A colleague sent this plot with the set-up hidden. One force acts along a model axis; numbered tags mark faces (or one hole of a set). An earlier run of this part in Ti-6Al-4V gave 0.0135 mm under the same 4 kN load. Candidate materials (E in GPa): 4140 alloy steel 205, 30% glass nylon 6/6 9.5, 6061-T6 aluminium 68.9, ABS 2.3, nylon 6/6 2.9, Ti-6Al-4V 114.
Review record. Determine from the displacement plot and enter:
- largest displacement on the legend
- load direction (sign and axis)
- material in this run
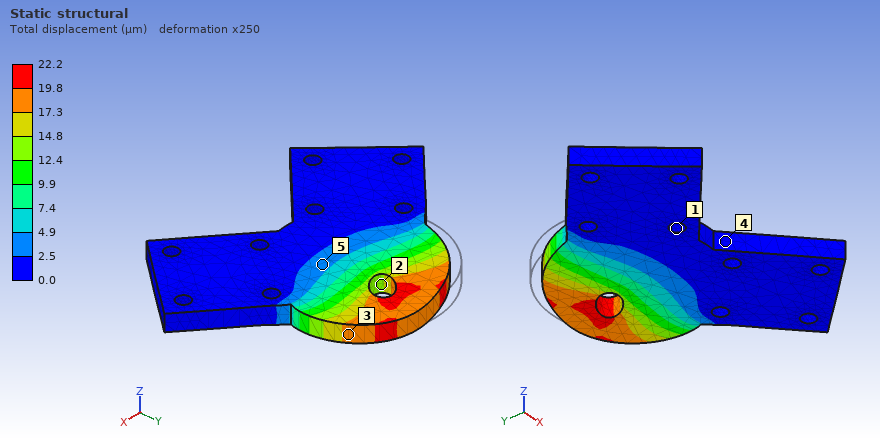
22.2 µm
+X
6061-T6 aluminium
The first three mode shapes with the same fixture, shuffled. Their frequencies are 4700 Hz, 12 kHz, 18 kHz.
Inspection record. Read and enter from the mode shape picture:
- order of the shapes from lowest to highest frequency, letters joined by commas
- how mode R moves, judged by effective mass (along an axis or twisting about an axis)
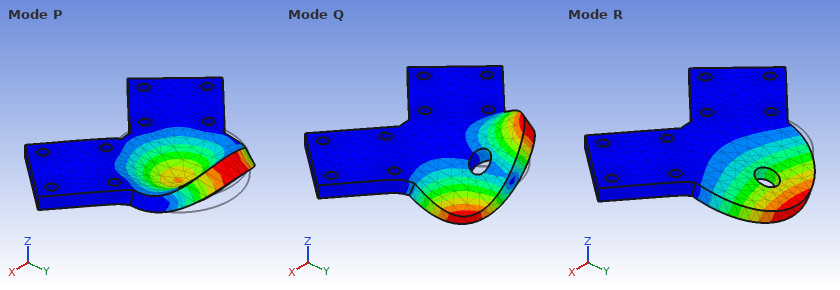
R, Q, P
along Z
